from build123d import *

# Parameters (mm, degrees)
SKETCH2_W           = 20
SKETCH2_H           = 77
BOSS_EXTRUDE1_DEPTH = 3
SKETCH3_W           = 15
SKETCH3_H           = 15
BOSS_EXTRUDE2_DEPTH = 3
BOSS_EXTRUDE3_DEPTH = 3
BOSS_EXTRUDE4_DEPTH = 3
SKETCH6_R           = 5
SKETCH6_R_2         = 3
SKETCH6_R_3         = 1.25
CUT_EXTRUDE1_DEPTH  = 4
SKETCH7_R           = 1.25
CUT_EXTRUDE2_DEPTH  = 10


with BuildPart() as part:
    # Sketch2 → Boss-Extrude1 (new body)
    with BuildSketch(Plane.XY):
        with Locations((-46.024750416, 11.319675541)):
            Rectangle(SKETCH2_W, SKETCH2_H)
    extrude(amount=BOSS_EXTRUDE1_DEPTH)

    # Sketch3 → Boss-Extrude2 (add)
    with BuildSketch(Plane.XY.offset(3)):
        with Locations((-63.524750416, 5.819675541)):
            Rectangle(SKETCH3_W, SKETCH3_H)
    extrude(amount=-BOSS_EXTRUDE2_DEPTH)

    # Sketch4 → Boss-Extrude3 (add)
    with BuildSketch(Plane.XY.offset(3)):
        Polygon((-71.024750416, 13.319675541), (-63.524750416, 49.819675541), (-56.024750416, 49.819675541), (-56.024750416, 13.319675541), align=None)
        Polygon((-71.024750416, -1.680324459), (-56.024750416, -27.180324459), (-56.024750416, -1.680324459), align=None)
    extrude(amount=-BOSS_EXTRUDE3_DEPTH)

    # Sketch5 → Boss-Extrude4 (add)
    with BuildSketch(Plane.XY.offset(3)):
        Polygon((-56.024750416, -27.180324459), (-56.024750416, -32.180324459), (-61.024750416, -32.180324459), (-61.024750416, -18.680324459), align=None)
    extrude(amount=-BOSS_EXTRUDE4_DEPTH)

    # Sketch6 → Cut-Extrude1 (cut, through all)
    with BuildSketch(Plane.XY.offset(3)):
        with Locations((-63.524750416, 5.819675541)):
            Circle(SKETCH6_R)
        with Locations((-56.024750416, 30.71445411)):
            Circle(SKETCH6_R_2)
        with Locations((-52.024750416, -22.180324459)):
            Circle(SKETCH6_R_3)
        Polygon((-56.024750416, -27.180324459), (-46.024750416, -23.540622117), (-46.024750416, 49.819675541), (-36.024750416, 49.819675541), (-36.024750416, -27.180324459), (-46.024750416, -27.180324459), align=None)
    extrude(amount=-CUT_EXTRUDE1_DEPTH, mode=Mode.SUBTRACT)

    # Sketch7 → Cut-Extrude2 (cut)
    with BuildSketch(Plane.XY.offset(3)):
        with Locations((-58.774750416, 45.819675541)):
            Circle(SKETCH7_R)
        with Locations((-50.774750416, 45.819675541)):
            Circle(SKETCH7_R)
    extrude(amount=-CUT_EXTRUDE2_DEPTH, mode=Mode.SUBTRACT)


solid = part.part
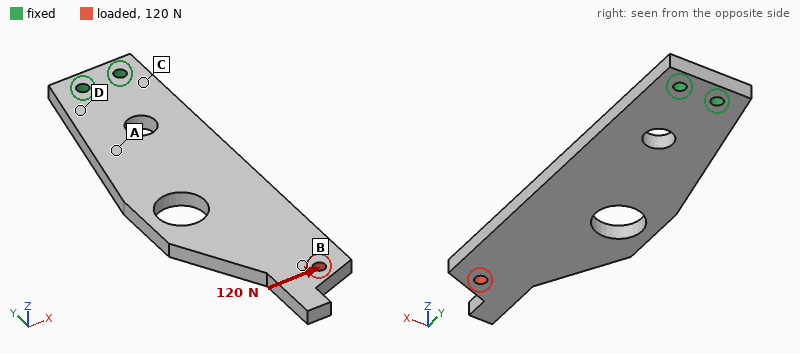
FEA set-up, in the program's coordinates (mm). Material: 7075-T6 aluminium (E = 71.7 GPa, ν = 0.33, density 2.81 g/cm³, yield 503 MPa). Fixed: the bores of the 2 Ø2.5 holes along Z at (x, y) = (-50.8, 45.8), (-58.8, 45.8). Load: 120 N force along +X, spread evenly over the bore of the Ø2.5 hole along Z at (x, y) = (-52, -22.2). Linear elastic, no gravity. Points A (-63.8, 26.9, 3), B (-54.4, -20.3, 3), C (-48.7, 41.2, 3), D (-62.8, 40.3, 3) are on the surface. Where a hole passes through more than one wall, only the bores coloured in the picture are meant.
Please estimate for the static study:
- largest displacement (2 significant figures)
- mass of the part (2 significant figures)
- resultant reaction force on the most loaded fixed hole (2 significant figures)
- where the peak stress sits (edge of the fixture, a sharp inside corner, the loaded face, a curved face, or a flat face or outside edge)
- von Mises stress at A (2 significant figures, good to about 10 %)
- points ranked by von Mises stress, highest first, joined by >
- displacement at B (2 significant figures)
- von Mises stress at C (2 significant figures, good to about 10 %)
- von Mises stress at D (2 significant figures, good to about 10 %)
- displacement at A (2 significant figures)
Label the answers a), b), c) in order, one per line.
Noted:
a) 0.14 mm
b) 13 g
c) 830 N
d) edge of the fixture
e) 14 MPa
f) C > D > A > B
g) 0.11 mm
h) 34 MPa
i) 28 MPa
j) 0.023 mm
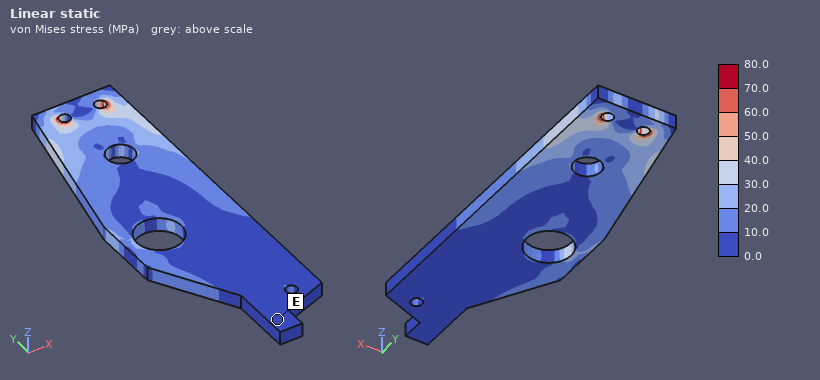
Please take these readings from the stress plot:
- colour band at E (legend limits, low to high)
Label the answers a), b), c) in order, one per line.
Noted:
a) 0.0 to 10.0 MPa
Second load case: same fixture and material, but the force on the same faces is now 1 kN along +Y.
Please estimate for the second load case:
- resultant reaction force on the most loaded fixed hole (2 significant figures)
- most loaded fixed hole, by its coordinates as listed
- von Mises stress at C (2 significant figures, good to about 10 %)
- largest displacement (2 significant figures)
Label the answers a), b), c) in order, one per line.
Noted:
a) 790 N
b) (-50.8, 45.8)
c) 35 MPa
d) 86 µm
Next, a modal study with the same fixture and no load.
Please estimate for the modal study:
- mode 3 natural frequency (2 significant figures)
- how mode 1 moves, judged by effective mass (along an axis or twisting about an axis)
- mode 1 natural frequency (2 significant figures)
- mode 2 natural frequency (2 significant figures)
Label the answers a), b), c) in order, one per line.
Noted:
a) 2600 Hz
b) along Z
c) 470 Hz
d) 2600 Hz
